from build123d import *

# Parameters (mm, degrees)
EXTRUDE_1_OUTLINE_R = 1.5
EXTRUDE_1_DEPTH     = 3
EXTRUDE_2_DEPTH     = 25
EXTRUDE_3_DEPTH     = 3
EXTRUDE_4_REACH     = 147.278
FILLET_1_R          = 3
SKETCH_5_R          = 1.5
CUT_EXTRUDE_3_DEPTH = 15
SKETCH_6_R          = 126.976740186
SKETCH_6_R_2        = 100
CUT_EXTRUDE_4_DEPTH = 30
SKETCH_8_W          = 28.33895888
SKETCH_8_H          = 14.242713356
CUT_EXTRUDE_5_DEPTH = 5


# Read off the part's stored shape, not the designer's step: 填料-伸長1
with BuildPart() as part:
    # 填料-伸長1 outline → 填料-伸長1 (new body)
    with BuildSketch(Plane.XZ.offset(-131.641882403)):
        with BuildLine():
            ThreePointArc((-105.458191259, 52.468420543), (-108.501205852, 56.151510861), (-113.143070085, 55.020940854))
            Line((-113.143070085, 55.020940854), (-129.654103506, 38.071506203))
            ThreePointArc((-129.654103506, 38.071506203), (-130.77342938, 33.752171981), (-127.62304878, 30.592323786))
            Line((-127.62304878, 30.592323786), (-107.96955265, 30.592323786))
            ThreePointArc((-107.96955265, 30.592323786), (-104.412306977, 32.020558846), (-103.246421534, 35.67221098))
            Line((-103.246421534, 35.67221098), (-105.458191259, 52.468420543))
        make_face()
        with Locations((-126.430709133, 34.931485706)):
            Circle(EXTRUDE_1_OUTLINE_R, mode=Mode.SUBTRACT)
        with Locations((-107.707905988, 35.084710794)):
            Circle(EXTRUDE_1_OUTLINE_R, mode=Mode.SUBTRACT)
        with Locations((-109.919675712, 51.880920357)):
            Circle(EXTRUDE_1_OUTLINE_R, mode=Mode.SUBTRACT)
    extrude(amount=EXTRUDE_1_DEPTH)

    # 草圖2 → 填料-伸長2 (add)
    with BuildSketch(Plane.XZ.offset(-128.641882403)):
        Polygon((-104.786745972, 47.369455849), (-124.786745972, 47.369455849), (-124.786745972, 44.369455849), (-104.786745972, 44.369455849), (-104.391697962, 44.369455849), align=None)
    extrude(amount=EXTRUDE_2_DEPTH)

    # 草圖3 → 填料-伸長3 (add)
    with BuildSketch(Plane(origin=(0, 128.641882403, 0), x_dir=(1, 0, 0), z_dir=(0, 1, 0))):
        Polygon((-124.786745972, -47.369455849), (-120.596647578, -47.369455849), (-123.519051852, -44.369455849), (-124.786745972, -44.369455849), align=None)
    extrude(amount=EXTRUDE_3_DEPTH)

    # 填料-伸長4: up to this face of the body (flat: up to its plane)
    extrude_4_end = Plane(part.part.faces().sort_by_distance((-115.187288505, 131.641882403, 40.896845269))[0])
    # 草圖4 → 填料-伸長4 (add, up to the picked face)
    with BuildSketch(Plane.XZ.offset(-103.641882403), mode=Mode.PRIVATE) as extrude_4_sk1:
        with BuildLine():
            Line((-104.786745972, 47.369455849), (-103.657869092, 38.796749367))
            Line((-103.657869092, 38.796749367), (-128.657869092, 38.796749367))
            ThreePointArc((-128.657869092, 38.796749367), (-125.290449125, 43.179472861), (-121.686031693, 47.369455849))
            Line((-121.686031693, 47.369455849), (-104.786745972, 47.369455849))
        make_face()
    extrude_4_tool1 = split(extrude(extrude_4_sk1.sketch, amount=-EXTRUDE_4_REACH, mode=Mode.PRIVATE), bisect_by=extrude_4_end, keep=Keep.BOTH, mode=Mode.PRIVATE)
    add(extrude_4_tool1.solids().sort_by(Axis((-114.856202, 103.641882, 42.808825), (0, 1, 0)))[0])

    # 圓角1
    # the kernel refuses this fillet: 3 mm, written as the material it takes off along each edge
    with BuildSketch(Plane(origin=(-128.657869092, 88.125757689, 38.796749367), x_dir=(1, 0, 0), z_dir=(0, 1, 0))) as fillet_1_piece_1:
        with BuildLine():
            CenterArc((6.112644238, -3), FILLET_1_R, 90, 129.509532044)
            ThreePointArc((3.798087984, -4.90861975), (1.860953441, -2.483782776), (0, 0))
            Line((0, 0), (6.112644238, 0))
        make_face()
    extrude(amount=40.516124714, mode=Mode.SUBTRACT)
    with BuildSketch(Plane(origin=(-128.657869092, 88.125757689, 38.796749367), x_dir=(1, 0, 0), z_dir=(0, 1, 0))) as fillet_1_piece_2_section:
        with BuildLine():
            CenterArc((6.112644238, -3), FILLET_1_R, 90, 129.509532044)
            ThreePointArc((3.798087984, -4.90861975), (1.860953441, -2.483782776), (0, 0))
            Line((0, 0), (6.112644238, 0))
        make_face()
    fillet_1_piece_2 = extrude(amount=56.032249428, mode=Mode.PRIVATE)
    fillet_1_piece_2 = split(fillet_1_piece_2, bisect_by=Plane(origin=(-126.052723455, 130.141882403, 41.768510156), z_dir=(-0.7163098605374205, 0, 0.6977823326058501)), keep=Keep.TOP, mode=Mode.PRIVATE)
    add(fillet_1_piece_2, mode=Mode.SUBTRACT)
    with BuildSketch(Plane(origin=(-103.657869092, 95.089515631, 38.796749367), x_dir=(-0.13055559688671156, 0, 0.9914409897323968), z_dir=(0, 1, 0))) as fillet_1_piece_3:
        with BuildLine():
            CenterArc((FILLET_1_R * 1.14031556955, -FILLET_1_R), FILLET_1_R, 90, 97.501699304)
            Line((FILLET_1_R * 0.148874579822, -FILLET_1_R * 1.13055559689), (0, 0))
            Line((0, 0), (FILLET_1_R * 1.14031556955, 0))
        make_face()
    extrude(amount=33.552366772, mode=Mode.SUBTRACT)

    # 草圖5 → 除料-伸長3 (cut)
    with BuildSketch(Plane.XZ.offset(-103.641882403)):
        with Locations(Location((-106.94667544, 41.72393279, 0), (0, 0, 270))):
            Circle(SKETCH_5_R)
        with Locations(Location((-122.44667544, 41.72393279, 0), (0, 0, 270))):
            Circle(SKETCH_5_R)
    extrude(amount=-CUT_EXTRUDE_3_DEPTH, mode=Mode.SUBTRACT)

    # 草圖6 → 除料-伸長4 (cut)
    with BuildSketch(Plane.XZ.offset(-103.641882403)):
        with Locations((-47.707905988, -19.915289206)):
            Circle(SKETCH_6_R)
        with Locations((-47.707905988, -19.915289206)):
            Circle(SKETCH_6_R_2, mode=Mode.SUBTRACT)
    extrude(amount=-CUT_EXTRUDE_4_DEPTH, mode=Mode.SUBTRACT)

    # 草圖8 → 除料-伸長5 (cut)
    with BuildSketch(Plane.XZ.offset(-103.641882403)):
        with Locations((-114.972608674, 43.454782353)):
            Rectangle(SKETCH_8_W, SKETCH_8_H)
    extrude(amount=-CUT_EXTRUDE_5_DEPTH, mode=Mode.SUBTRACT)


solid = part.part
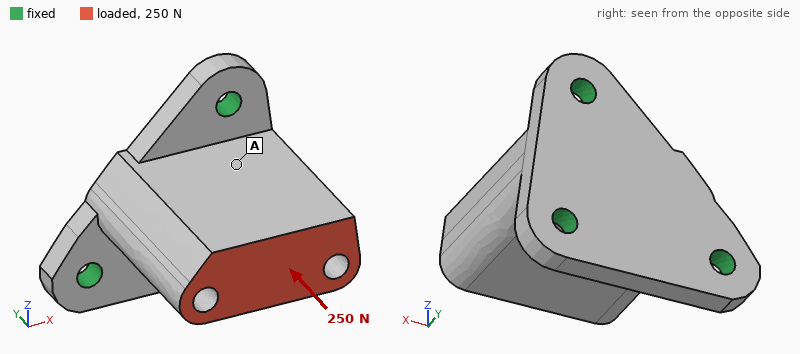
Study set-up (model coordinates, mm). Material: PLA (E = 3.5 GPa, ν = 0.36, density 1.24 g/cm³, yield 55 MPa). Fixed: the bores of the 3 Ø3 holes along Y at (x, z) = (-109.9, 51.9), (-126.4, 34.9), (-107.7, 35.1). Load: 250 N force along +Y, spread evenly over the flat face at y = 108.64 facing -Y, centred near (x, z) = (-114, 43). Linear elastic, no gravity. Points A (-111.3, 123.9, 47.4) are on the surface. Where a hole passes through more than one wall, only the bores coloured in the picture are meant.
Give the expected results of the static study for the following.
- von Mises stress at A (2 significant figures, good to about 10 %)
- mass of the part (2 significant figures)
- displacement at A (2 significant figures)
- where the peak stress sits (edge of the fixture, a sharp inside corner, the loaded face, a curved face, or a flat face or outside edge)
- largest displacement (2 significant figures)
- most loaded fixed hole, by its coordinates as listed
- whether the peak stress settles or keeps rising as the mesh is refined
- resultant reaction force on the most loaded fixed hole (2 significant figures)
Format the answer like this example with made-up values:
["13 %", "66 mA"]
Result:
["2.8 MPa", "5.8 g", "37 µm", "edge of the fixture", "80 µm", "(-109.9, 51.9)", "keeps rising", "120 N"]
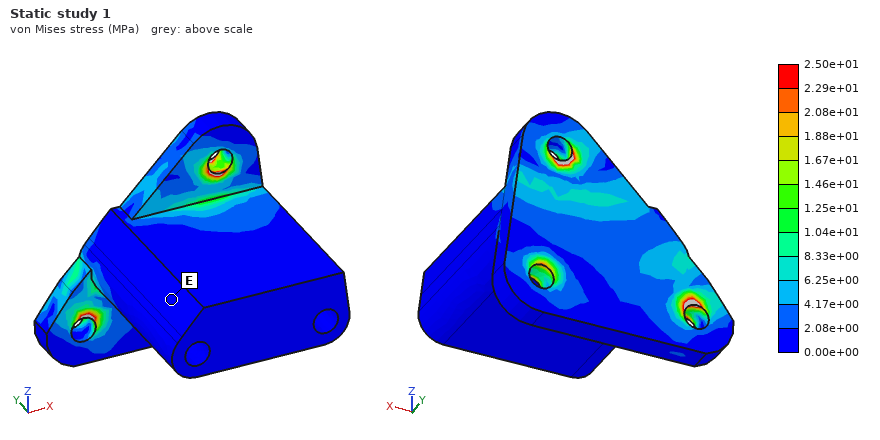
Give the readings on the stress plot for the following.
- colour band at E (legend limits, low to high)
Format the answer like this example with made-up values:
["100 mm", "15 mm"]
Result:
["0.00e+00 to 2.08e+00 MPa"]
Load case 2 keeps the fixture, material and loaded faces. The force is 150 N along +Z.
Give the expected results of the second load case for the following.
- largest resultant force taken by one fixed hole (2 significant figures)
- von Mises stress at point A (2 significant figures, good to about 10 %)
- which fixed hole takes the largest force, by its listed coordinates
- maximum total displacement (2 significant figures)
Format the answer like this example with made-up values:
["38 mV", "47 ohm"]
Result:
["250 N", "12 MPa", "(-109.9, 51.9)", "0.39 mm"]
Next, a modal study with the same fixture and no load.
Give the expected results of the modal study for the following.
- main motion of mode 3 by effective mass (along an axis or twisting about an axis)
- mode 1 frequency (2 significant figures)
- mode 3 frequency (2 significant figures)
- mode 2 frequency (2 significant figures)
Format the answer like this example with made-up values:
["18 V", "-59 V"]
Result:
["along Y", "2700 Hz", "6800 Hz", "3600 Hz"]
